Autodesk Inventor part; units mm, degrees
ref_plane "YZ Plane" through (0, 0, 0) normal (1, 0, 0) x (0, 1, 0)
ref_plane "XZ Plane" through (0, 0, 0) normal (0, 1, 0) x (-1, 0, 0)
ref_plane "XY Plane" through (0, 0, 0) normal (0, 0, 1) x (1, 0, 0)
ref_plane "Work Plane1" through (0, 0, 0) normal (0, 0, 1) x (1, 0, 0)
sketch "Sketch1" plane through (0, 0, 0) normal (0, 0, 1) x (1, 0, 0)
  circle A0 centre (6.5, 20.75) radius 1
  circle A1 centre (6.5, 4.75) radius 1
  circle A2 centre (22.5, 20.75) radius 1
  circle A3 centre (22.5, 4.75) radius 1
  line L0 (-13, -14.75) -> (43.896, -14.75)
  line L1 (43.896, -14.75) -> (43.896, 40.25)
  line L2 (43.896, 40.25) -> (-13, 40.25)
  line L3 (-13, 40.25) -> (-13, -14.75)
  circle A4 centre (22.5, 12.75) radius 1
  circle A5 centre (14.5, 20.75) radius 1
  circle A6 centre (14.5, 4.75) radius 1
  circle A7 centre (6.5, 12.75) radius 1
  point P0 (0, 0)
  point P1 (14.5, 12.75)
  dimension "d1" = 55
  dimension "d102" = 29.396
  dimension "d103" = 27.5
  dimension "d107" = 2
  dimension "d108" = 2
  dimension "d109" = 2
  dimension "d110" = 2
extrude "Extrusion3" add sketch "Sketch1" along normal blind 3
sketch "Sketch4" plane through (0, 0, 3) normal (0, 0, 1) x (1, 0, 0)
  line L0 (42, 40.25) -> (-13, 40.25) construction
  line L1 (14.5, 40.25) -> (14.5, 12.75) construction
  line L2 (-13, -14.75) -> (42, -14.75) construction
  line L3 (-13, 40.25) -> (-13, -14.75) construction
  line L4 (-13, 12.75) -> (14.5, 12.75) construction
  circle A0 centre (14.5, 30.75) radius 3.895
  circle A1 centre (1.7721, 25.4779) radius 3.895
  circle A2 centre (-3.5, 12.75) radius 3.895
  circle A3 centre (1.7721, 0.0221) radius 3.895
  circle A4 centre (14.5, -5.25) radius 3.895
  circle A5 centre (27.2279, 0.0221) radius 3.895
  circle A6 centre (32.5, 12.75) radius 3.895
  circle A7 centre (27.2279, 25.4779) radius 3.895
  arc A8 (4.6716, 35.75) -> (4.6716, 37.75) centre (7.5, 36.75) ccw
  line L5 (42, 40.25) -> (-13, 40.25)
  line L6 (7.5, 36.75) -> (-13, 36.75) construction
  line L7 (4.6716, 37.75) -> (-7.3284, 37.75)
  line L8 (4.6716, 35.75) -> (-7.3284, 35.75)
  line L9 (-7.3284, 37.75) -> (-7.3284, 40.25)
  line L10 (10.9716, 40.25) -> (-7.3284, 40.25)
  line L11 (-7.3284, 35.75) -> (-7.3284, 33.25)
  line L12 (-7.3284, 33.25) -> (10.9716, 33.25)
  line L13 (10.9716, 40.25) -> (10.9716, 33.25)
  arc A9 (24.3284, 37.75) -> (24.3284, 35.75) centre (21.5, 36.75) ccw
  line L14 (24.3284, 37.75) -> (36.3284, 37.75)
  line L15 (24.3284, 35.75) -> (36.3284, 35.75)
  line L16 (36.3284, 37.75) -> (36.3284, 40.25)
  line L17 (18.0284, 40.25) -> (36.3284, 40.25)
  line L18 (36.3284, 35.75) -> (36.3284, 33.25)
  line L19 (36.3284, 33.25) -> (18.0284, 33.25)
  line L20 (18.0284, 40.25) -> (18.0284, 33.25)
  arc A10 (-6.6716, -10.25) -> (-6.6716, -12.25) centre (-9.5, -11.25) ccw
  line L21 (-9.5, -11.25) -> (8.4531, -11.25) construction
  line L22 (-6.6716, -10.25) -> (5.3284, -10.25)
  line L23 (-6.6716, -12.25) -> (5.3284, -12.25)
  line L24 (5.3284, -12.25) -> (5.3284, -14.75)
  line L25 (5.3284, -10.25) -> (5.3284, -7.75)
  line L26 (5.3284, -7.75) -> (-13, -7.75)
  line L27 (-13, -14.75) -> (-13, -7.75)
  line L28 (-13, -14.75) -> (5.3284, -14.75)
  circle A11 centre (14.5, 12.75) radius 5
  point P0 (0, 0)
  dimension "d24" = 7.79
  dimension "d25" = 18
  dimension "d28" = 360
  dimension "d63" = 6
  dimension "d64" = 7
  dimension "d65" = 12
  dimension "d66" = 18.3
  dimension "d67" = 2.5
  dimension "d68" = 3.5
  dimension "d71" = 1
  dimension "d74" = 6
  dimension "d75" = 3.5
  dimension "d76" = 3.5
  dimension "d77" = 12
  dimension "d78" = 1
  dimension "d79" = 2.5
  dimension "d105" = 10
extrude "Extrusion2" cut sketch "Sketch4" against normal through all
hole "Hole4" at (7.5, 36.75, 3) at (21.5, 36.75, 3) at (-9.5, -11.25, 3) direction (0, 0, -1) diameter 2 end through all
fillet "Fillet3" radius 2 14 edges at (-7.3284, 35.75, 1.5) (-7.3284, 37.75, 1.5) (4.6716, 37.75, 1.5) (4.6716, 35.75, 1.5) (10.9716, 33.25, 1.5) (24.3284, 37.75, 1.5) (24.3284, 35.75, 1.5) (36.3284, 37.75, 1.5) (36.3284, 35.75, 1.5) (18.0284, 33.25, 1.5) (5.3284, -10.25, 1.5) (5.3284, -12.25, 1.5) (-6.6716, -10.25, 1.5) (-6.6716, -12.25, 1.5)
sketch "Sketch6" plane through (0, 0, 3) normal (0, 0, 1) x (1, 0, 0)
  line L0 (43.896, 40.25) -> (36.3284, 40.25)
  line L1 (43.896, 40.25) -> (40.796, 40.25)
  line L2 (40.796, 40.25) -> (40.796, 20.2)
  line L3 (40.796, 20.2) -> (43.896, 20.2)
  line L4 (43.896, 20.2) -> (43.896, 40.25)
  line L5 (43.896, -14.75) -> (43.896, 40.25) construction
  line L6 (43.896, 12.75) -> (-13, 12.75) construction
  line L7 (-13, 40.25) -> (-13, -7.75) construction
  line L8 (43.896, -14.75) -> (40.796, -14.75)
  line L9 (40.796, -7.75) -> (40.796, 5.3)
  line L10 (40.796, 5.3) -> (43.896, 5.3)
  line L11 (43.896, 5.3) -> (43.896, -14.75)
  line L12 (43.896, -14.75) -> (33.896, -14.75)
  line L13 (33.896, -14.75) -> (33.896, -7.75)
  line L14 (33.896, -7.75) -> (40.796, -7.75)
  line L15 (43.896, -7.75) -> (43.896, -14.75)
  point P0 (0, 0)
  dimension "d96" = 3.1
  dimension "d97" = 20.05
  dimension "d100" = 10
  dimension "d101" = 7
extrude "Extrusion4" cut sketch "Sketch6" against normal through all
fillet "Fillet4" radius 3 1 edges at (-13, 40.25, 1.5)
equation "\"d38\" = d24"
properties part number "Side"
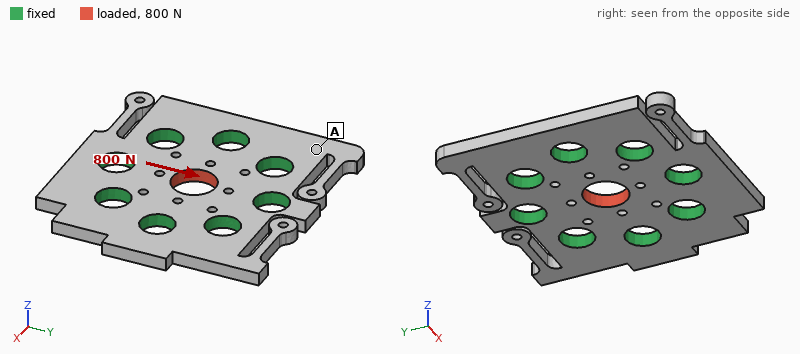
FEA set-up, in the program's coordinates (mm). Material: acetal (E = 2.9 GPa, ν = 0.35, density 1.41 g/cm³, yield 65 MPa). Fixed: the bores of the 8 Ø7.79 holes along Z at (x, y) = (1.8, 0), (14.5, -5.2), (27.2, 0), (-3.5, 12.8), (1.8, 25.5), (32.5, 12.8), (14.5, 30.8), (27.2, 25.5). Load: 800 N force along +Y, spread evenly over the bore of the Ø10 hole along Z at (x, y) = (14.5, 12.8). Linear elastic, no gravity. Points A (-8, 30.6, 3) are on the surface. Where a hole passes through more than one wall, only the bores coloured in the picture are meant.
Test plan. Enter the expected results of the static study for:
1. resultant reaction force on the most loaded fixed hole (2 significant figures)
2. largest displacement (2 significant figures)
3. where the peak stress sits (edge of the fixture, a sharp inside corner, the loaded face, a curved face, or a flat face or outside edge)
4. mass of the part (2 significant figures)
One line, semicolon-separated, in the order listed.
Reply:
190 N; 30 µm; a curved face; 9.5 g
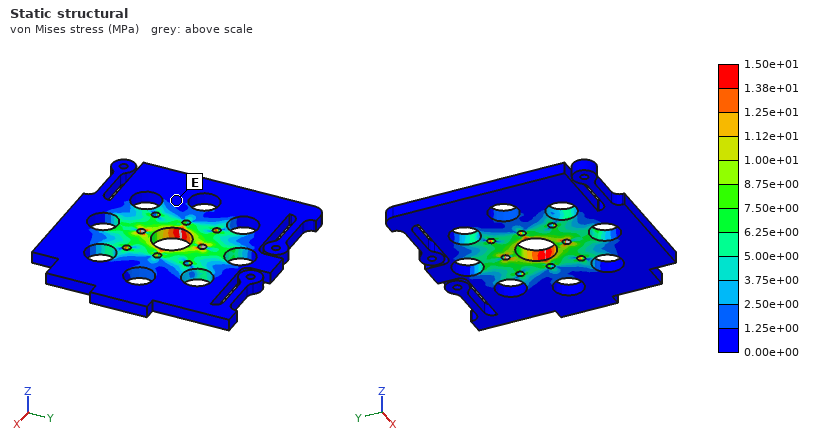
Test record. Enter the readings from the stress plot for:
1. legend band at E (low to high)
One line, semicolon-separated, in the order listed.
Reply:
0.00e+00 to 1.25e+00 MPa
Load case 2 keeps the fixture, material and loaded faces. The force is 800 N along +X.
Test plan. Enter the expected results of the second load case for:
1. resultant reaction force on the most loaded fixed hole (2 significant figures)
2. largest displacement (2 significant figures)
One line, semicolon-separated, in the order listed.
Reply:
190 N; 30 µm
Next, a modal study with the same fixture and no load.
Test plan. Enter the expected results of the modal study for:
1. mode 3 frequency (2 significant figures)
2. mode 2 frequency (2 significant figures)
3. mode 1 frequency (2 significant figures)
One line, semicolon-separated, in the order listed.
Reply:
1100 Hz; 1100 Hz; 1000 Hz
